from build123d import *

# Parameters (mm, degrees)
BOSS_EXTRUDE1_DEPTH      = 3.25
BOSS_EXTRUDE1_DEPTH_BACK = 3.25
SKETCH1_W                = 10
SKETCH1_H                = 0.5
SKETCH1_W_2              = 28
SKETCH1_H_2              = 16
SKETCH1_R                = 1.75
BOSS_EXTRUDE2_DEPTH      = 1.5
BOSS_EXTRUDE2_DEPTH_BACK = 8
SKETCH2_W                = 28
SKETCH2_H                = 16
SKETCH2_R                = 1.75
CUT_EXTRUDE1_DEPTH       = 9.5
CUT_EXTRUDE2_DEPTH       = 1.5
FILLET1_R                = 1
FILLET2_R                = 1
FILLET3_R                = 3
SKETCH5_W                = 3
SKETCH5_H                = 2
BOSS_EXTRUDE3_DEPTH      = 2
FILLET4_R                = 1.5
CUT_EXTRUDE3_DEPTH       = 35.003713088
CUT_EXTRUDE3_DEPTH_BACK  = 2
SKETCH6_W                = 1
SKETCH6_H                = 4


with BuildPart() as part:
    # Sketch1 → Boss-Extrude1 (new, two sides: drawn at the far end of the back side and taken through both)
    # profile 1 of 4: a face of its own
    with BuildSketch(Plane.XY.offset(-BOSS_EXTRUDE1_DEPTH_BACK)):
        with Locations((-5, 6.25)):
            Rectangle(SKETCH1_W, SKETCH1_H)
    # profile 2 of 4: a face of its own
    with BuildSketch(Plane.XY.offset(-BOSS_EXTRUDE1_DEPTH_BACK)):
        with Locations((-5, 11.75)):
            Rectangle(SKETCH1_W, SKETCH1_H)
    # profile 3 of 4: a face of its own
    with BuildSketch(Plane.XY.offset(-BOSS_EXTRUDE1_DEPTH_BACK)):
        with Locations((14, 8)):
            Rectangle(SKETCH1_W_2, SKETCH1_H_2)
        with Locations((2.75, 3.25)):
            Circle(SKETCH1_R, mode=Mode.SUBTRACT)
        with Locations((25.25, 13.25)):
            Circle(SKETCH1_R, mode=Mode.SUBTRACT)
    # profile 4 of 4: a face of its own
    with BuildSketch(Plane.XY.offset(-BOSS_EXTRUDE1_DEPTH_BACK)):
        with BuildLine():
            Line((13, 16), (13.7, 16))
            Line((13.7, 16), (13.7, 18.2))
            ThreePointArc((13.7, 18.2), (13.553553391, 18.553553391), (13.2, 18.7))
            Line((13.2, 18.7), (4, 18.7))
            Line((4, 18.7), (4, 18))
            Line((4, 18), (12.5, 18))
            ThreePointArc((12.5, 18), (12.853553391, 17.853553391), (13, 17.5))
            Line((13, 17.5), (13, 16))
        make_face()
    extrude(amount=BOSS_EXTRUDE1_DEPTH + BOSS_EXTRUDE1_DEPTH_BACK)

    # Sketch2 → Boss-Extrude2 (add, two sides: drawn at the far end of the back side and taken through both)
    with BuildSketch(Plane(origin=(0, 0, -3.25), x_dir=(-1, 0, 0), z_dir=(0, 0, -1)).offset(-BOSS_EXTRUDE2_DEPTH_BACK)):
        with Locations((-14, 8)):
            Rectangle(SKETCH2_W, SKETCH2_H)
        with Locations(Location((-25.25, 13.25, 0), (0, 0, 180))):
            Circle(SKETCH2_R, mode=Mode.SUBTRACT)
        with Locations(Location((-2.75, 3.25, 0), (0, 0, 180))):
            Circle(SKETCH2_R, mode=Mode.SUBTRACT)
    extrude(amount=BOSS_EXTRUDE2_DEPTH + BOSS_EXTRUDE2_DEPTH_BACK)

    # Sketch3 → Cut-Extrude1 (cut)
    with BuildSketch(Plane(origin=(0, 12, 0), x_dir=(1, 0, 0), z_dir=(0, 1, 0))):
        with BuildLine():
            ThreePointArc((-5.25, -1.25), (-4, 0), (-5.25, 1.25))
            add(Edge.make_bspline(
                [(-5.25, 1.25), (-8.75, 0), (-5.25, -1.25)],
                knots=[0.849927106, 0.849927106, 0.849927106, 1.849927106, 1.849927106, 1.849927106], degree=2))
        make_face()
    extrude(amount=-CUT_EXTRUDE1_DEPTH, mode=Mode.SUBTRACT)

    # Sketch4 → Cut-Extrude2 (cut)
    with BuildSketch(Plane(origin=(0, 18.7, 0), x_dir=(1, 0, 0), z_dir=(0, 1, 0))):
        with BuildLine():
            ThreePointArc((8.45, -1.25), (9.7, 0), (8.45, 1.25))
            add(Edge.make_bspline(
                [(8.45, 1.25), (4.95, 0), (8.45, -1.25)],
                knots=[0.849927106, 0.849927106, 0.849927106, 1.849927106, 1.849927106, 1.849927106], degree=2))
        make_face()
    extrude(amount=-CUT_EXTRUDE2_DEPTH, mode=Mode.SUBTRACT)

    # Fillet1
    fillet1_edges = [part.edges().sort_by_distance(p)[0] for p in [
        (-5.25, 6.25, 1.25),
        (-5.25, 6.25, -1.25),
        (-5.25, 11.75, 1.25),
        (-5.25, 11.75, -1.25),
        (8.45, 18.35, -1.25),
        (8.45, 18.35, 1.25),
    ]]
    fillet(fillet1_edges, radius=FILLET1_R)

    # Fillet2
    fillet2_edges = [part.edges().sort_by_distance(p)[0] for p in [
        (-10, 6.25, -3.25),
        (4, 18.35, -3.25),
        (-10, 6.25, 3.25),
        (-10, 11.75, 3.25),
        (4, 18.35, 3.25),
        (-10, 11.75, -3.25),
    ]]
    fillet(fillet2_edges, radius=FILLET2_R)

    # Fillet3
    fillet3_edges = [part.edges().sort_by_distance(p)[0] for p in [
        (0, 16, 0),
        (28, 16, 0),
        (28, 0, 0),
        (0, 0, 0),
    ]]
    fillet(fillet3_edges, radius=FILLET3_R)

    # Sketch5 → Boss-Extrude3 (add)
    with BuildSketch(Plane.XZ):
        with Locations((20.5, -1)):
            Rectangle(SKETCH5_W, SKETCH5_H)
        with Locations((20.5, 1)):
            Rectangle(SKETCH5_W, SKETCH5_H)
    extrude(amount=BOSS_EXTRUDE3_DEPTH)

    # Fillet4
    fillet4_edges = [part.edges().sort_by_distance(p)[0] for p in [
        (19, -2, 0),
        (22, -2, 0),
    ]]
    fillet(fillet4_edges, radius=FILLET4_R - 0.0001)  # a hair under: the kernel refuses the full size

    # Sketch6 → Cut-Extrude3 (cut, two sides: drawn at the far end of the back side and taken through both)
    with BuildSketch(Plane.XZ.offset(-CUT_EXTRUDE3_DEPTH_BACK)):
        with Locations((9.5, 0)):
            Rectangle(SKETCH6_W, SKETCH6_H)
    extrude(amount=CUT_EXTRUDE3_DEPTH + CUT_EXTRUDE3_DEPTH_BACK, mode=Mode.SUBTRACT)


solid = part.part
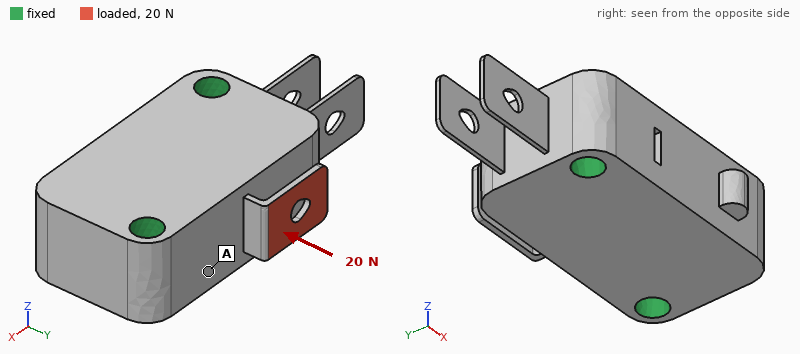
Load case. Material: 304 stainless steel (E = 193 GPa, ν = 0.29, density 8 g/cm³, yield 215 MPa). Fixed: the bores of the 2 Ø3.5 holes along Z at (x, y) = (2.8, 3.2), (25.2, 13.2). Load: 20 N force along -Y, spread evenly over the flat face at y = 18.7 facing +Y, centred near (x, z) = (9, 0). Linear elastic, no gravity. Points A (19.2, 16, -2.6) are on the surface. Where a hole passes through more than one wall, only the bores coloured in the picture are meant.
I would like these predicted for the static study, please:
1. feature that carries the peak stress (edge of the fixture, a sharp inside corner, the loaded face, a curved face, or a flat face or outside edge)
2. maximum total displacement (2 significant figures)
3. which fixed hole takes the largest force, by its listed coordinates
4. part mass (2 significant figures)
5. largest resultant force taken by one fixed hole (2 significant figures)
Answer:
a curved face
0.10 mm
(2.8, 3.2)
33 g
16 N
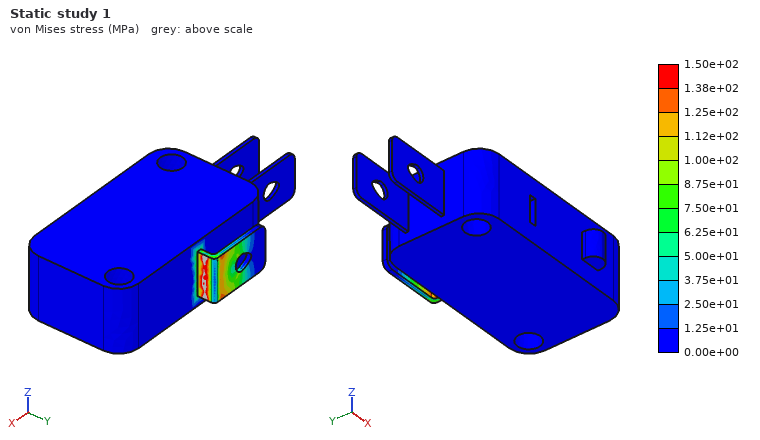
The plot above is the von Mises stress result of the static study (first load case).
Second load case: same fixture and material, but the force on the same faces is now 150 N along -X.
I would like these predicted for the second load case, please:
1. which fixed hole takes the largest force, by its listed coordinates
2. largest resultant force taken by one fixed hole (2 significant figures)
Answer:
(25.2, 13.2)
110 N
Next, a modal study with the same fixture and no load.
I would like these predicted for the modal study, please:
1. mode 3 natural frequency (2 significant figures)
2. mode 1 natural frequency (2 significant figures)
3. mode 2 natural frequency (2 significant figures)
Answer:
4900 Hz
4000 Hz
4000 Hz
